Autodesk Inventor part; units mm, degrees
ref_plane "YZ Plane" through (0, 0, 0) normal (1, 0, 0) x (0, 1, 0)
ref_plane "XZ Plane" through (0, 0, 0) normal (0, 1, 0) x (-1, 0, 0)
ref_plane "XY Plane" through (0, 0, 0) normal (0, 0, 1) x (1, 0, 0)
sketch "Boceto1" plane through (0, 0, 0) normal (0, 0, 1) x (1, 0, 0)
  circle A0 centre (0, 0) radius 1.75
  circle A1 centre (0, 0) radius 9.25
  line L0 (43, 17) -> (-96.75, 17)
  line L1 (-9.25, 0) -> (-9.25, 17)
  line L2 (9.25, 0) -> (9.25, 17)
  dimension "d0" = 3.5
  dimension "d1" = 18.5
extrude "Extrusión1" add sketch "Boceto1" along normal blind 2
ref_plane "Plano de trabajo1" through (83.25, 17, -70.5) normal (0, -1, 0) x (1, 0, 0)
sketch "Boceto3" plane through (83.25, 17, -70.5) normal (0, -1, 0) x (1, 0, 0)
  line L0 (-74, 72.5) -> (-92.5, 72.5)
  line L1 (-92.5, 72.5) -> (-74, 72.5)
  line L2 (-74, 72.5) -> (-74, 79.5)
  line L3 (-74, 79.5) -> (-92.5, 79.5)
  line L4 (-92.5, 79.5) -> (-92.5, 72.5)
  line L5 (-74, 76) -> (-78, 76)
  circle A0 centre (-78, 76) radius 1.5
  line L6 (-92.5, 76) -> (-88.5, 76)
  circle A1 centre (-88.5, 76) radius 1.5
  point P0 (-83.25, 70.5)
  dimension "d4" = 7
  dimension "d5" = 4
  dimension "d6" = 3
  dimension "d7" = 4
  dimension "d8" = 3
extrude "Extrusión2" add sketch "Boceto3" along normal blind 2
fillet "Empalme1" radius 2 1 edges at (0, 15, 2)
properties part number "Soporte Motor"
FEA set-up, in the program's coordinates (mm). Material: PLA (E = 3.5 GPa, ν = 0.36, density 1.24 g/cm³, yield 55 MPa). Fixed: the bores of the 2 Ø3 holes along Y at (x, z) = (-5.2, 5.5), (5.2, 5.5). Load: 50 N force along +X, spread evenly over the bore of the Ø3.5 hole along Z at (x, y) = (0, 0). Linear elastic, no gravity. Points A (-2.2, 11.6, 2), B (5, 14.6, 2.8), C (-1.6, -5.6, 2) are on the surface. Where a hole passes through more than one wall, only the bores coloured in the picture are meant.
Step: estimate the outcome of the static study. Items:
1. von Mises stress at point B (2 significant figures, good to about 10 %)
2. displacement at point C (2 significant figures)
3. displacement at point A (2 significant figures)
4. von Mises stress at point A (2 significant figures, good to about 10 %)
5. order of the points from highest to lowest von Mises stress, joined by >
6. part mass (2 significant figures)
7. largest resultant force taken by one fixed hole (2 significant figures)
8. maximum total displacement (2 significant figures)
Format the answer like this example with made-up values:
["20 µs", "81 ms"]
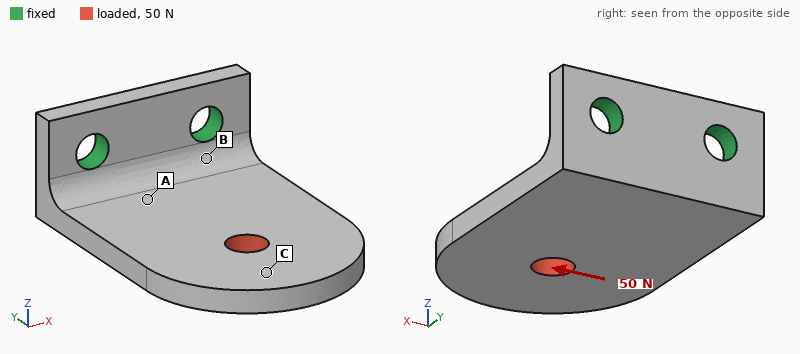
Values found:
["15 MPa", "0.20 mm", "0.044 mm", "8.2 MPa", "B > A > C", "1.4 g", "71 N", "0.22 mm"]
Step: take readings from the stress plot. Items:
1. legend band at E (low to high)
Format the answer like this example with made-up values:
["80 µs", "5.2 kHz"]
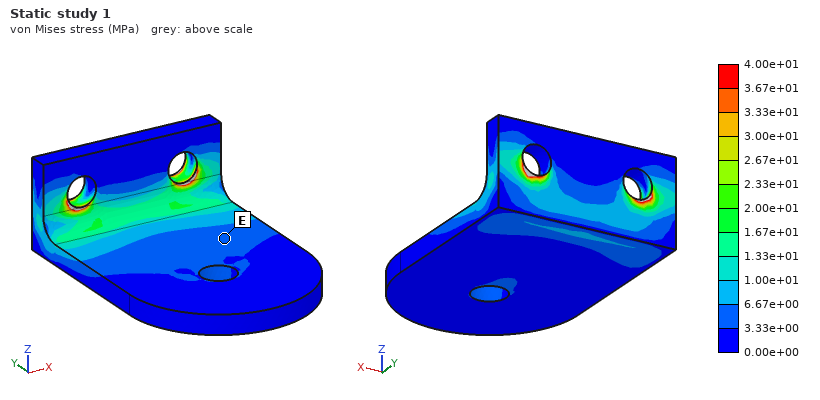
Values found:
["3.33e+00 to 6.67e+00 MPa"]
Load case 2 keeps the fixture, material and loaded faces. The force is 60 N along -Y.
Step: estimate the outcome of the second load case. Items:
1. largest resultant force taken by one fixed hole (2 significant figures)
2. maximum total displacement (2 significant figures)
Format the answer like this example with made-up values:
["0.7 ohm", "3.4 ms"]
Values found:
["30 N", "0.23 mm"]
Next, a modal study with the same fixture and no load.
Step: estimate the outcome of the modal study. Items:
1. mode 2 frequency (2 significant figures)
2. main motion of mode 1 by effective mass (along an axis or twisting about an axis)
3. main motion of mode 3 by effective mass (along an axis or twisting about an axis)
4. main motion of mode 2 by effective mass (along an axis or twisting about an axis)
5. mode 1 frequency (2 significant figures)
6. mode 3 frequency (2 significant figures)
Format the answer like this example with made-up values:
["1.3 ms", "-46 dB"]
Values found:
["2800 Hz", "along Z", "along X", "along X", "930 Hz", "3800 Hz"]
